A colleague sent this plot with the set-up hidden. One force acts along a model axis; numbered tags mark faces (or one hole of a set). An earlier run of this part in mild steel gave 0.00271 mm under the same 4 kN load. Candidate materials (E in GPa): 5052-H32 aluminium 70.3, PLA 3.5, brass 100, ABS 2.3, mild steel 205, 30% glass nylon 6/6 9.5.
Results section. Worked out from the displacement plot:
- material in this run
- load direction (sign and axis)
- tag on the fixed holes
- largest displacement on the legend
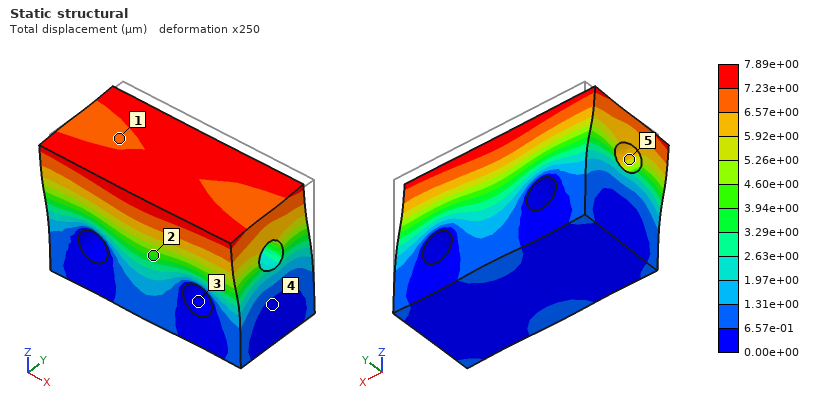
5052-H32 aluminium
-Y
3
7.89e+00 µm
